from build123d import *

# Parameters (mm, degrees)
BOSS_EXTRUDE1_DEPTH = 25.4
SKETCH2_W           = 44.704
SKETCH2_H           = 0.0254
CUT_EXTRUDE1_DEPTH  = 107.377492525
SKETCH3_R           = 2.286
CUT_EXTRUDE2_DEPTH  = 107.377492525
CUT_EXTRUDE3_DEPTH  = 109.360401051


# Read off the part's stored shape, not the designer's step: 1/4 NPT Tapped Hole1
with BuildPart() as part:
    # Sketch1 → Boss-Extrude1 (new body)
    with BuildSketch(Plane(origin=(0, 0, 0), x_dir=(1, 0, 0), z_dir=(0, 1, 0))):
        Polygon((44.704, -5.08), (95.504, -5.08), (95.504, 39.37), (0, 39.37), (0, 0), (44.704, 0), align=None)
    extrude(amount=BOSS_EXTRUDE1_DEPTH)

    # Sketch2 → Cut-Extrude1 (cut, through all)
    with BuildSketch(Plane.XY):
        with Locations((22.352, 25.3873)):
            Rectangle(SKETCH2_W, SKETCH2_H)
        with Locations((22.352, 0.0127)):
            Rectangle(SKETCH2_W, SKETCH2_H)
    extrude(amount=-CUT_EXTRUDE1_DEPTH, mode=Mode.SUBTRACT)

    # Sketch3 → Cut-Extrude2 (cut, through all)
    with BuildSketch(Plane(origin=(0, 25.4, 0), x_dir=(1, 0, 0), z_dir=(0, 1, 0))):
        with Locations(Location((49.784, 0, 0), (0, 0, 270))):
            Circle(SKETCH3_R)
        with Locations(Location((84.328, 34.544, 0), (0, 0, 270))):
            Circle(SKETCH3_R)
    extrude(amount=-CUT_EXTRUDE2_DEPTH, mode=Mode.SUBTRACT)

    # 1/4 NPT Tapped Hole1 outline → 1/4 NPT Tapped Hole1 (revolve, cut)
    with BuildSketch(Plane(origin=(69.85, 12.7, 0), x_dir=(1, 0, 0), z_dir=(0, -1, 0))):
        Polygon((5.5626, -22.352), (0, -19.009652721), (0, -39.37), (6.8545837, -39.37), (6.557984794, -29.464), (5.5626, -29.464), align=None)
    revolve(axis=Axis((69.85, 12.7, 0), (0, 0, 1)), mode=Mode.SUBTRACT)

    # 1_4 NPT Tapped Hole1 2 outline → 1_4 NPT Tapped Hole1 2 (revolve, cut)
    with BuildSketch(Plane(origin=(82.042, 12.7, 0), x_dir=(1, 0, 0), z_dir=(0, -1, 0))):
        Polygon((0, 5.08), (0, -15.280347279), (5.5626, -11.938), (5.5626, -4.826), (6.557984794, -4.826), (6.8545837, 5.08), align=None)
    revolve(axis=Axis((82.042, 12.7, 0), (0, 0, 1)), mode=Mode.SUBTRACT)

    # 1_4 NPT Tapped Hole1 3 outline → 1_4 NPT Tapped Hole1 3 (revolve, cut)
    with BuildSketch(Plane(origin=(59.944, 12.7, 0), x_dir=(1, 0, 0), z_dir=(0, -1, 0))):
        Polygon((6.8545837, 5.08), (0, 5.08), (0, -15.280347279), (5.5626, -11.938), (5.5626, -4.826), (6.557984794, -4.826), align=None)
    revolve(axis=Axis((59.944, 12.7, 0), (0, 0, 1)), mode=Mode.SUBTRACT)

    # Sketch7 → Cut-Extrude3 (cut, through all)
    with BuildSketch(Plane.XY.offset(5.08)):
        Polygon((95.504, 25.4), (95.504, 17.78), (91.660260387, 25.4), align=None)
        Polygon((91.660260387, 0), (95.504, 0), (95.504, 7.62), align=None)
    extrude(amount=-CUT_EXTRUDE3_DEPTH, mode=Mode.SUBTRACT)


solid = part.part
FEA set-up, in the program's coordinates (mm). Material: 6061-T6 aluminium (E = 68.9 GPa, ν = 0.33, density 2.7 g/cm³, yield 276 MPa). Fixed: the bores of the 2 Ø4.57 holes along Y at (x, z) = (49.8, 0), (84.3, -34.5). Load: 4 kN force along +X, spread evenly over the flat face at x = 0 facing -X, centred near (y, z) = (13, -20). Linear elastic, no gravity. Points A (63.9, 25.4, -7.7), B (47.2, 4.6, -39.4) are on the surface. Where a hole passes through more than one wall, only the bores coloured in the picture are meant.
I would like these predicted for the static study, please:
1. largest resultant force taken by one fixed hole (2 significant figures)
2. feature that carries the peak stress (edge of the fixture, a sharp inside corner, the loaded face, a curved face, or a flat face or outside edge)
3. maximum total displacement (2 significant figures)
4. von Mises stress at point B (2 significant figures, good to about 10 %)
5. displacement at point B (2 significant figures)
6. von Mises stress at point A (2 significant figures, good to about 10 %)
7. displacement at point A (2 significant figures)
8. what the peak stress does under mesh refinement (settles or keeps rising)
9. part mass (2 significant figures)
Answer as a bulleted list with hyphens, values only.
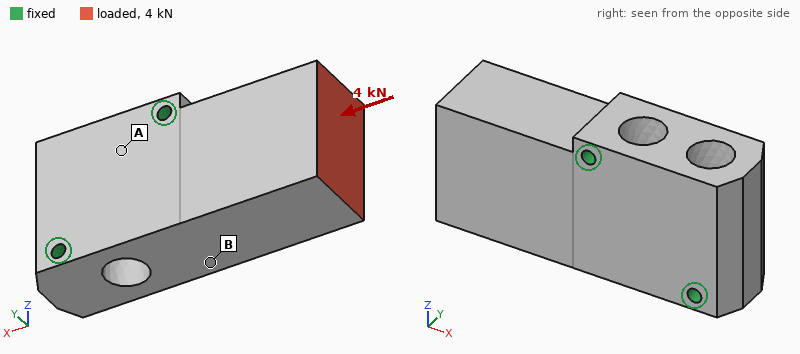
- 2.1 kN
- edge of the fixture
- 9.9 µm
- 5.4 MPa
- 4.8 µm
- 2.0 MPa
- 1.6 µm
- keeps rising
- 250 g
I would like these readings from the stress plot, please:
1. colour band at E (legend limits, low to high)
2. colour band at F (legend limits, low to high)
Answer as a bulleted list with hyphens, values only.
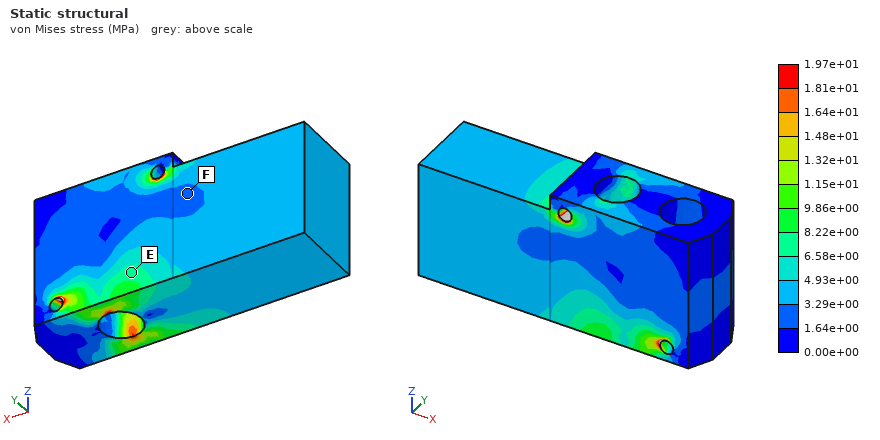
- 6.58e+00 to 8.22e+00 MPa
- 1.64e+00 to 3.29e+00 MPa
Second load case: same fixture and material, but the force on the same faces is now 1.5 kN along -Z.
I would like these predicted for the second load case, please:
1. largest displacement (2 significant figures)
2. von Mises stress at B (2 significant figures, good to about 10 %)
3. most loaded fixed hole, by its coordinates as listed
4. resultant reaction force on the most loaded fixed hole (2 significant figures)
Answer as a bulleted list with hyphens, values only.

- 19 µm
- 8.7 MPa
- (49.8, 0)
- 2.6 kN
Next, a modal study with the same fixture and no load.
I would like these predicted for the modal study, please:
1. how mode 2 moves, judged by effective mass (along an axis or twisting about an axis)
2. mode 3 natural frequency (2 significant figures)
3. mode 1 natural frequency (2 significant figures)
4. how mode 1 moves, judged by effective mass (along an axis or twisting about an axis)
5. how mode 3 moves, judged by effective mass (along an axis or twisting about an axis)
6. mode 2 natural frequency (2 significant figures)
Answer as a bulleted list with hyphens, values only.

- along Z
- 9500 Hz
- 4500 Hz
- along Y
- twisting about X
- 6700 Hz
